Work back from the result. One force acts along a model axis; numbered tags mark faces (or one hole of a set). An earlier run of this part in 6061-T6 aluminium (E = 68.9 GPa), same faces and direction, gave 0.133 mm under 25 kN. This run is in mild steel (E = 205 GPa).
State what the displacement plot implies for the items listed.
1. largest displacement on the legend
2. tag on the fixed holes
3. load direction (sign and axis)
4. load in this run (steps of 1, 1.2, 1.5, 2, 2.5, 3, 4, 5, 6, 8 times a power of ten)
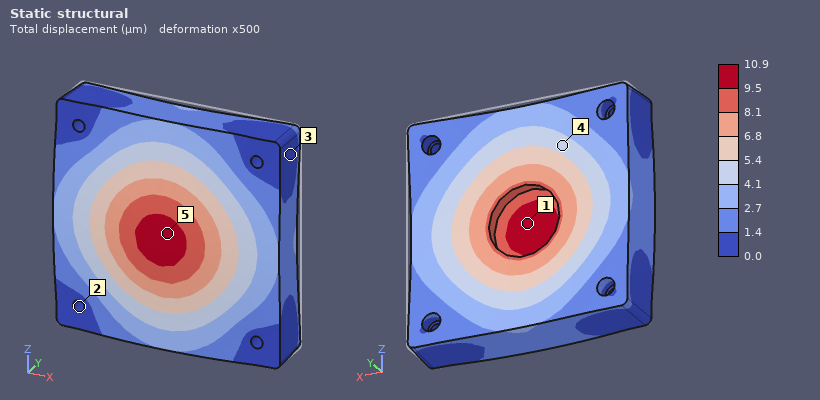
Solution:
10.9 µm
2
-Y
6 kN
